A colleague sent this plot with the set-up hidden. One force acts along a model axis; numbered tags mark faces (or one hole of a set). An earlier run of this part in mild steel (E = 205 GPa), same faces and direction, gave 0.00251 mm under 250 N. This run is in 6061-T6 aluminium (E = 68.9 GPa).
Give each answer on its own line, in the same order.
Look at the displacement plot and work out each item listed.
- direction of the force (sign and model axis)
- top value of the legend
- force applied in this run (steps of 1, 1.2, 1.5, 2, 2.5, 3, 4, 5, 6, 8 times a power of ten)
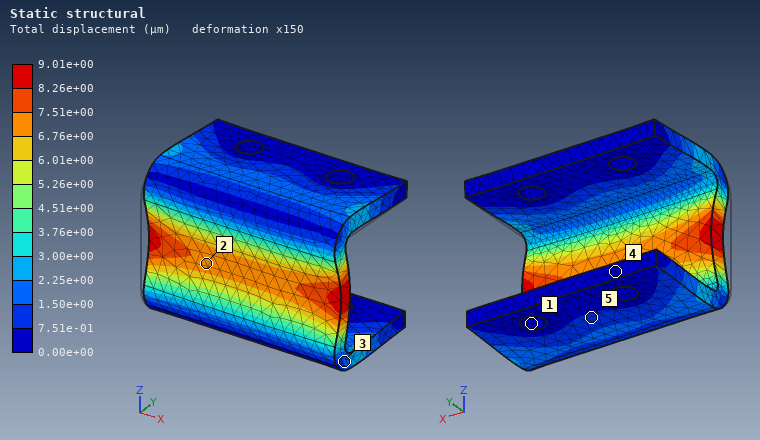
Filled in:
+Y
9.01e+00 µm
300 N
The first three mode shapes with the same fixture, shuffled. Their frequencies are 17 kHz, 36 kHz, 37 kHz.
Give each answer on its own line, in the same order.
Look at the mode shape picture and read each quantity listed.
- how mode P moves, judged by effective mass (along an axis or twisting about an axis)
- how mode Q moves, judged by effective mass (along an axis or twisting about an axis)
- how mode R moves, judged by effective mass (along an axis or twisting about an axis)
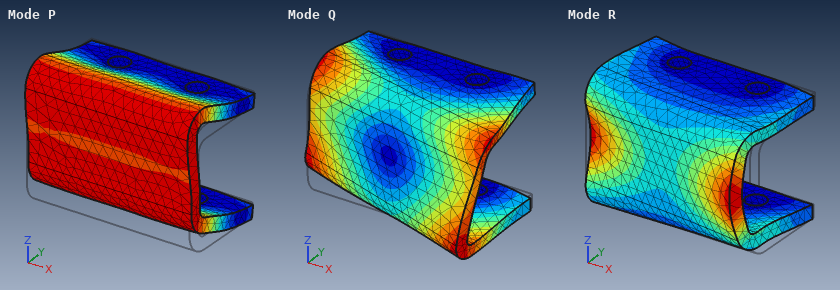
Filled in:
along Z
twisting about Y
along X
